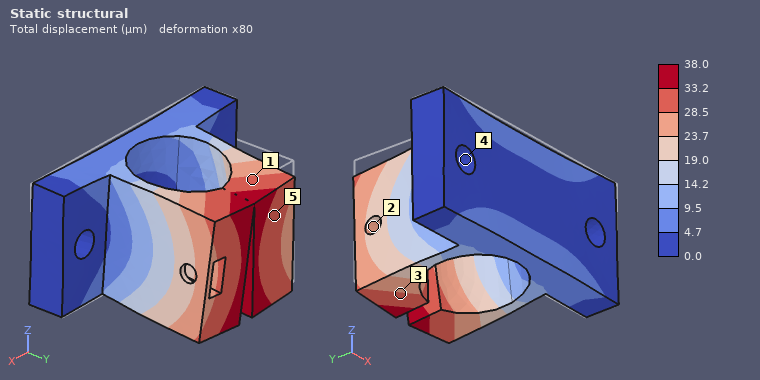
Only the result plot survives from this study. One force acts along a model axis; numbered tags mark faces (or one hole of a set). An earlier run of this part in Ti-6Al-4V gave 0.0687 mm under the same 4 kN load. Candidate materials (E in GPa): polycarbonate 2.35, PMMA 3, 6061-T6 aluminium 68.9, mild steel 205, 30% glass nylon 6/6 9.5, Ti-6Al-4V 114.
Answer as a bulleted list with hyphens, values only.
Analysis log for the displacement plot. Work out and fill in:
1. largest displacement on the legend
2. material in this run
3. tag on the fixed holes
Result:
- 38.0 µm
- mild steel
- 4
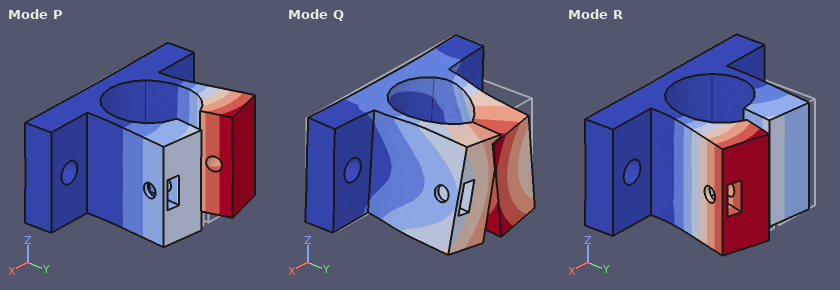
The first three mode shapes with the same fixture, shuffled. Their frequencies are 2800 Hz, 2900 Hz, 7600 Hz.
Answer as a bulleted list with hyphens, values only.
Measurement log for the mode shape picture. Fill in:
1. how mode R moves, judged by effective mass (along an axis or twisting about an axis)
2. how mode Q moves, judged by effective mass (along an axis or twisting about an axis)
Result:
- along X
- along Z
